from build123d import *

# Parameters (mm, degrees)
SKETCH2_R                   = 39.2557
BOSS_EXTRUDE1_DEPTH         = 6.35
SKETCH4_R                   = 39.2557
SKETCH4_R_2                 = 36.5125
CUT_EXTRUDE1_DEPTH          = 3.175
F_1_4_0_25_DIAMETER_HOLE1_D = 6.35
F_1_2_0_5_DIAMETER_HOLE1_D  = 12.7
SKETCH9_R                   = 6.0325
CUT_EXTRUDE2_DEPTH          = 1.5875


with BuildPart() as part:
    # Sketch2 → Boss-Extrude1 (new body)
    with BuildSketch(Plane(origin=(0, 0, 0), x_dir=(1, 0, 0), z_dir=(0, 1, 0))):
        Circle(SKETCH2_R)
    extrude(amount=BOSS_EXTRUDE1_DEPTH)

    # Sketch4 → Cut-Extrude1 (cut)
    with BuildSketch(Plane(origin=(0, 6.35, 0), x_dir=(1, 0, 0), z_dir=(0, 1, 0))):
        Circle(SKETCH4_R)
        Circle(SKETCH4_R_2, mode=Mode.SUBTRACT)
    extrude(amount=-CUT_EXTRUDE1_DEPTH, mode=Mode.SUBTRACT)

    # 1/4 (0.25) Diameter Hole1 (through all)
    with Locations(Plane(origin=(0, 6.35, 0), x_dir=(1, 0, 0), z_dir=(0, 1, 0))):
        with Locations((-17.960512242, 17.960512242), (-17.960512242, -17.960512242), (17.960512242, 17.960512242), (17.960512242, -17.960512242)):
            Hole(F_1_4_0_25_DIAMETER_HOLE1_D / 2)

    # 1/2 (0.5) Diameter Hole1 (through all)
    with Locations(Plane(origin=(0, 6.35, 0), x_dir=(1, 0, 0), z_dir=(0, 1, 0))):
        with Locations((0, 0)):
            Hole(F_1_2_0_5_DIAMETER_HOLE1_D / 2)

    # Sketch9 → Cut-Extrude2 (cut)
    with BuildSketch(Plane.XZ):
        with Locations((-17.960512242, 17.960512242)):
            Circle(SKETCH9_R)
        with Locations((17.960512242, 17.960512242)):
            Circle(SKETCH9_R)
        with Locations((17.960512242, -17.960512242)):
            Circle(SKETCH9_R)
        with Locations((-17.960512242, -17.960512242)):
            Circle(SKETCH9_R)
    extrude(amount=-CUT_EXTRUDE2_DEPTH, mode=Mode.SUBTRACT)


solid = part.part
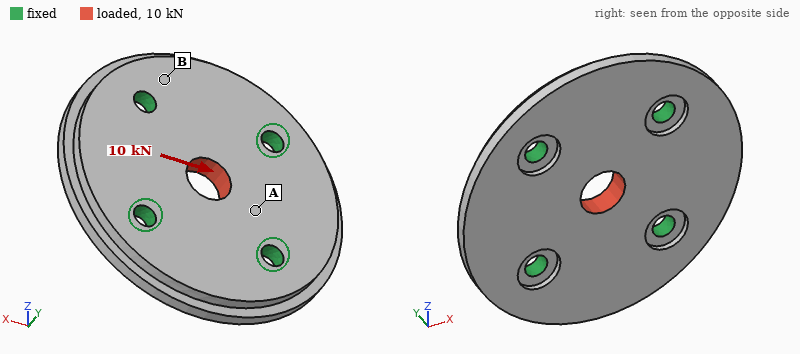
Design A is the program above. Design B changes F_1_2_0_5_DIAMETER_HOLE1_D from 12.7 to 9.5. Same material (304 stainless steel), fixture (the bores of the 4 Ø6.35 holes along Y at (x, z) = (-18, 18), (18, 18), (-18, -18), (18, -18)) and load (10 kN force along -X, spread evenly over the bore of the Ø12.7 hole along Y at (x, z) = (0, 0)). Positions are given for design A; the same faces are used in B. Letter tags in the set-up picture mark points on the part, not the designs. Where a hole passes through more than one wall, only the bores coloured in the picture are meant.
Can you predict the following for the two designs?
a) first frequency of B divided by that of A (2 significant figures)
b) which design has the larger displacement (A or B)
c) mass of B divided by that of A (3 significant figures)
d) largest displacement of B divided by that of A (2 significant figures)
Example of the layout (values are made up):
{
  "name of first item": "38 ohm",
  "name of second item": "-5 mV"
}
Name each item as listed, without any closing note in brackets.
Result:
{
  "first frequency of B divided by that of A": "1.0",
  "which design has the larger displacement": "B",
  "mass of B divided by that of A": "1.01",
  "largest displacement of B divided by that of A": "1.1"
}
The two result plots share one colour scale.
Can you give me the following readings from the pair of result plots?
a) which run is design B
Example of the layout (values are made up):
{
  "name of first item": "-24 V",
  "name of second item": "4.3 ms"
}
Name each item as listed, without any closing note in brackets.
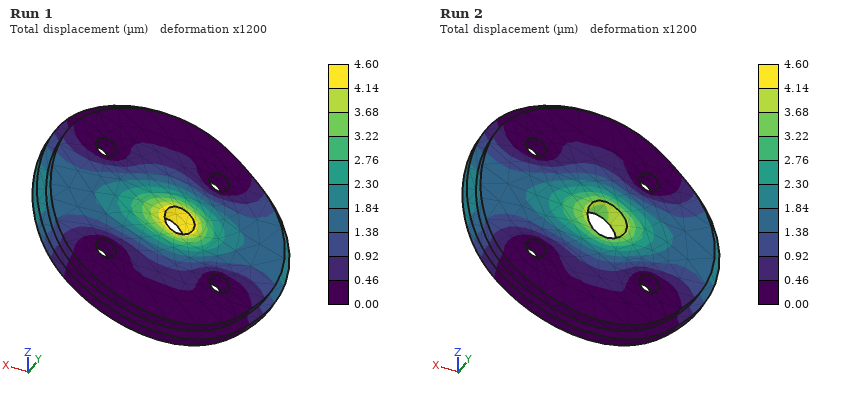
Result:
{
  "which run is design B": "Run 1"
}
